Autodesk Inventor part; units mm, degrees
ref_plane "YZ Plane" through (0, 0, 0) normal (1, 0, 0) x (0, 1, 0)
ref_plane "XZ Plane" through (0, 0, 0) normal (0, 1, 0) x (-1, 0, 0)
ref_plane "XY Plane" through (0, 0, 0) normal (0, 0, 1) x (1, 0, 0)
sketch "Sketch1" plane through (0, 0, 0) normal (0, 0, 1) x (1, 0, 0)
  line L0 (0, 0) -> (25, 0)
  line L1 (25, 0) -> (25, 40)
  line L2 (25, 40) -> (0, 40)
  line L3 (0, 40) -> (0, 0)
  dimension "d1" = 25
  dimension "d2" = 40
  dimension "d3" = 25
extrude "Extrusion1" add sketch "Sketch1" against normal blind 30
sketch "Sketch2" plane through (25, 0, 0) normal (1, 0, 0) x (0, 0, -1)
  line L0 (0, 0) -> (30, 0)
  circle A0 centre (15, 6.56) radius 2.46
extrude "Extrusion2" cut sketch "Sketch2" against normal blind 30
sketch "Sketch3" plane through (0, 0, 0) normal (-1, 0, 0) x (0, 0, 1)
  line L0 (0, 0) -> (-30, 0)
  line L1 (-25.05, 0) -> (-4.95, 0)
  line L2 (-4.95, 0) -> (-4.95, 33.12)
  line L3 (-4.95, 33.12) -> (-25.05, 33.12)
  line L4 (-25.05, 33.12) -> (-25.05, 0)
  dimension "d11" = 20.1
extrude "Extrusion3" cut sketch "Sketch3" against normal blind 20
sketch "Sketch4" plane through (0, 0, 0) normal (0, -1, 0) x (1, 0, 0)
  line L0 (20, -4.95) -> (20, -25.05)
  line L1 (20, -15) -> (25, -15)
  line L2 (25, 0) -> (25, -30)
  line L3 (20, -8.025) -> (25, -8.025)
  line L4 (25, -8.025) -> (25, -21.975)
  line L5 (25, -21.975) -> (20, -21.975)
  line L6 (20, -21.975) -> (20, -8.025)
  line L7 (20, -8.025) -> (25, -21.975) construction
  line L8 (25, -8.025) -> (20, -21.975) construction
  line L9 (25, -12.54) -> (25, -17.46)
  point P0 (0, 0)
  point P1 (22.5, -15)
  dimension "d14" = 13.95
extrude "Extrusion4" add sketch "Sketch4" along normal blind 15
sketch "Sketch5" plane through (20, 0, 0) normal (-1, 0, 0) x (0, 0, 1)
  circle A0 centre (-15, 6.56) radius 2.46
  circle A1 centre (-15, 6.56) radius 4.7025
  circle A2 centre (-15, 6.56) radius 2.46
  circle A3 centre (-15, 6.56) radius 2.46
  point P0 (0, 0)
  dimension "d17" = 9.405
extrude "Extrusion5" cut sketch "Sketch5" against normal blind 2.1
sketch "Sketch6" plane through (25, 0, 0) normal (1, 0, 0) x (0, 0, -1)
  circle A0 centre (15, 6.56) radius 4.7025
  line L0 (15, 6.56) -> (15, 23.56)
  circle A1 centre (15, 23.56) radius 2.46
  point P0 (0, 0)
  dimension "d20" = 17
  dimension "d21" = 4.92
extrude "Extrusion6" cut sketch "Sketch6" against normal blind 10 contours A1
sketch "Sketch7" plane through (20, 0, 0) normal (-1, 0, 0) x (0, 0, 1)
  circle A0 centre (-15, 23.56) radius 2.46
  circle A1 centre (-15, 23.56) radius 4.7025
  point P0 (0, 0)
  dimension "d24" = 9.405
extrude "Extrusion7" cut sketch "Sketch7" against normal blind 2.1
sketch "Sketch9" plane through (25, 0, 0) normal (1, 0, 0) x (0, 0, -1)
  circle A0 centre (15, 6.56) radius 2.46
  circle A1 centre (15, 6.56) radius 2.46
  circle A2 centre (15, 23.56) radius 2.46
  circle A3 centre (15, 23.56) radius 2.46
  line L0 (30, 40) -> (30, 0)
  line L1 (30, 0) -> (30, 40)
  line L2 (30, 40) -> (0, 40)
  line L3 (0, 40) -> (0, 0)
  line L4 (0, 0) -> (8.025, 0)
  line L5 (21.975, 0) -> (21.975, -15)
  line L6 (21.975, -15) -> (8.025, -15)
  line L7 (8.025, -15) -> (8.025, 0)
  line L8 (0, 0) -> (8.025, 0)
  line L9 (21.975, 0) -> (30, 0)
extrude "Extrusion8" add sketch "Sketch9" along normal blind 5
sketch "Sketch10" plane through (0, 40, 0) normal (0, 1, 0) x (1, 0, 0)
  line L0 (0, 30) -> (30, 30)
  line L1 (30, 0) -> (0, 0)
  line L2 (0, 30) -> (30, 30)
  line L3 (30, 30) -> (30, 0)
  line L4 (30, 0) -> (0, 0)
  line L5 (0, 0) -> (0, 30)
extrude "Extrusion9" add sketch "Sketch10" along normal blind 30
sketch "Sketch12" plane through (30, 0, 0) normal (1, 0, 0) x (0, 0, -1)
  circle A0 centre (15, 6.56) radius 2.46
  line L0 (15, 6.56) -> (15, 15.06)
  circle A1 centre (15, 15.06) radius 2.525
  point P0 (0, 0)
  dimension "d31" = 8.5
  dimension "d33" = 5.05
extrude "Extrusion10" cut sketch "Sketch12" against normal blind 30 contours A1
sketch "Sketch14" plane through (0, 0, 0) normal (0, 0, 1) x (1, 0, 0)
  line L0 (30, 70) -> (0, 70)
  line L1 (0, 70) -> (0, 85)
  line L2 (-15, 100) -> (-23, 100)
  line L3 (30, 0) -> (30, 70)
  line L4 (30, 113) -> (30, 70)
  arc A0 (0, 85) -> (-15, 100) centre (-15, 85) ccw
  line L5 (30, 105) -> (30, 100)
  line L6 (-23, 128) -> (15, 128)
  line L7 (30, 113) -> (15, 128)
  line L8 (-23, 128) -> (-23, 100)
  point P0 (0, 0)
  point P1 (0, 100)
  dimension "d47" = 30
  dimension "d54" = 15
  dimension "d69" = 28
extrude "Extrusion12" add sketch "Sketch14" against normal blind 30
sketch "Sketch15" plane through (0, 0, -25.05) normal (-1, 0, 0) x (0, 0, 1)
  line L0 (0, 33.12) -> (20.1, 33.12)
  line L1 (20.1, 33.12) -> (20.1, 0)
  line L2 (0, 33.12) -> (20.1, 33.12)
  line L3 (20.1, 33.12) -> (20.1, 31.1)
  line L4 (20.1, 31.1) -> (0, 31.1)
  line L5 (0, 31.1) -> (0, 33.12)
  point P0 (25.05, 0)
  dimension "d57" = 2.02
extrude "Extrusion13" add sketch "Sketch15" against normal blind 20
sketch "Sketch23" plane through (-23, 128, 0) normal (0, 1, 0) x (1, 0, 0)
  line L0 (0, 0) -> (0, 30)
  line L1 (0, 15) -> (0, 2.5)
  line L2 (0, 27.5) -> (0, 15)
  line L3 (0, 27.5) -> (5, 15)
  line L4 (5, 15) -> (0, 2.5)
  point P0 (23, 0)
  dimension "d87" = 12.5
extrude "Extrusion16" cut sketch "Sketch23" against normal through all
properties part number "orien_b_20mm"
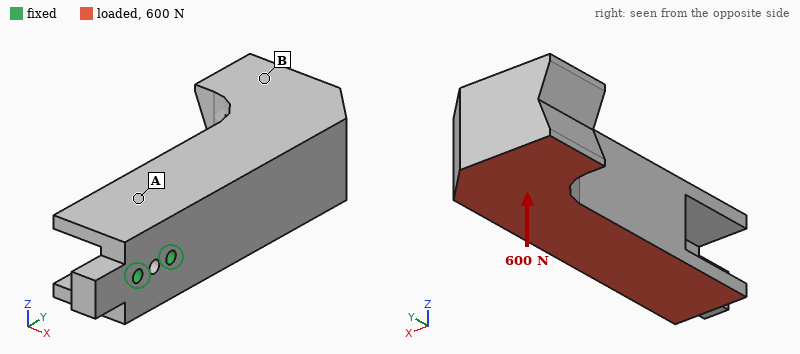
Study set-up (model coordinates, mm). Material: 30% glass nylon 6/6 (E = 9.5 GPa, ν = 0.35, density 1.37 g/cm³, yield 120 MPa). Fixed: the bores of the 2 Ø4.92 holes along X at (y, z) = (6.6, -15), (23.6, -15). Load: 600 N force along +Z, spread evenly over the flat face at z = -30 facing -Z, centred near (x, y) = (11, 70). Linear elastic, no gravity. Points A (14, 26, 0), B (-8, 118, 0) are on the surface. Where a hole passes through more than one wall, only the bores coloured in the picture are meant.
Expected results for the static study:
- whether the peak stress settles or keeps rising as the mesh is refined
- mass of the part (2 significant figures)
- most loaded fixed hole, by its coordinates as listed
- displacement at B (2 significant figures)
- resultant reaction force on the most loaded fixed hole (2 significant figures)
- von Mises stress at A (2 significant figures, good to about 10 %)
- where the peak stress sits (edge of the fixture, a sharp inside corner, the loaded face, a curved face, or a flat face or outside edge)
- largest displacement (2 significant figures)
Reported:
keeps rising
160 g
(23.6, -15)
0.46 mm
1.8 kN
8.5 MPa
edge of the fixture
0.54 mm
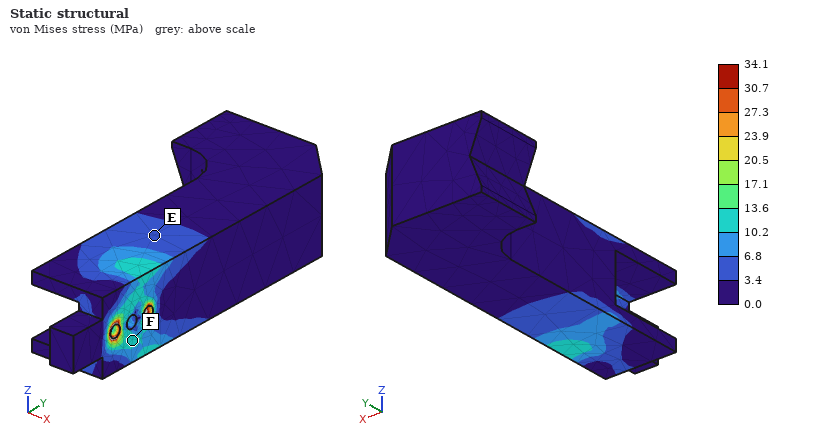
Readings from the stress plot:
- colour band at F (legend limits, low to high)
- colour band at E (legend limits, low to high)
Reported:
10.2 to 13.6 MPa
3.4 to 6.8 MPa
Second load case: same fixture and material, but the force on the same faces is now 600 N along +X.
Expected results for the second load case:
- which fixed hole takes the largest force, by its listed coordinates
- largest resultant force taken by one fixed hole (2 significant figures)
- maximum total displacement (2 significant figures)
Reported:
(23.6, -15)
1.7 kN
0.72 mm
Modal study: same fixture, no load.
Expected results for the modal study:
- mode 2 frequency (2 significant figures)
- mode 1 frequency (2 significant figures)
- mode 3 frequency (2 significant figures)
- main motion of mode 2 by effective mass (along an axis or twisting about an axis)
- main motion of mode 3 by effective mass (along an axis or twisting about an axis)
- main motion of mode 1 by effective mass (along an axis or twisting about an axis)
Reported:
510 Hz
430 Hz
1400 Hz
along Z
twisting about Y
along X
